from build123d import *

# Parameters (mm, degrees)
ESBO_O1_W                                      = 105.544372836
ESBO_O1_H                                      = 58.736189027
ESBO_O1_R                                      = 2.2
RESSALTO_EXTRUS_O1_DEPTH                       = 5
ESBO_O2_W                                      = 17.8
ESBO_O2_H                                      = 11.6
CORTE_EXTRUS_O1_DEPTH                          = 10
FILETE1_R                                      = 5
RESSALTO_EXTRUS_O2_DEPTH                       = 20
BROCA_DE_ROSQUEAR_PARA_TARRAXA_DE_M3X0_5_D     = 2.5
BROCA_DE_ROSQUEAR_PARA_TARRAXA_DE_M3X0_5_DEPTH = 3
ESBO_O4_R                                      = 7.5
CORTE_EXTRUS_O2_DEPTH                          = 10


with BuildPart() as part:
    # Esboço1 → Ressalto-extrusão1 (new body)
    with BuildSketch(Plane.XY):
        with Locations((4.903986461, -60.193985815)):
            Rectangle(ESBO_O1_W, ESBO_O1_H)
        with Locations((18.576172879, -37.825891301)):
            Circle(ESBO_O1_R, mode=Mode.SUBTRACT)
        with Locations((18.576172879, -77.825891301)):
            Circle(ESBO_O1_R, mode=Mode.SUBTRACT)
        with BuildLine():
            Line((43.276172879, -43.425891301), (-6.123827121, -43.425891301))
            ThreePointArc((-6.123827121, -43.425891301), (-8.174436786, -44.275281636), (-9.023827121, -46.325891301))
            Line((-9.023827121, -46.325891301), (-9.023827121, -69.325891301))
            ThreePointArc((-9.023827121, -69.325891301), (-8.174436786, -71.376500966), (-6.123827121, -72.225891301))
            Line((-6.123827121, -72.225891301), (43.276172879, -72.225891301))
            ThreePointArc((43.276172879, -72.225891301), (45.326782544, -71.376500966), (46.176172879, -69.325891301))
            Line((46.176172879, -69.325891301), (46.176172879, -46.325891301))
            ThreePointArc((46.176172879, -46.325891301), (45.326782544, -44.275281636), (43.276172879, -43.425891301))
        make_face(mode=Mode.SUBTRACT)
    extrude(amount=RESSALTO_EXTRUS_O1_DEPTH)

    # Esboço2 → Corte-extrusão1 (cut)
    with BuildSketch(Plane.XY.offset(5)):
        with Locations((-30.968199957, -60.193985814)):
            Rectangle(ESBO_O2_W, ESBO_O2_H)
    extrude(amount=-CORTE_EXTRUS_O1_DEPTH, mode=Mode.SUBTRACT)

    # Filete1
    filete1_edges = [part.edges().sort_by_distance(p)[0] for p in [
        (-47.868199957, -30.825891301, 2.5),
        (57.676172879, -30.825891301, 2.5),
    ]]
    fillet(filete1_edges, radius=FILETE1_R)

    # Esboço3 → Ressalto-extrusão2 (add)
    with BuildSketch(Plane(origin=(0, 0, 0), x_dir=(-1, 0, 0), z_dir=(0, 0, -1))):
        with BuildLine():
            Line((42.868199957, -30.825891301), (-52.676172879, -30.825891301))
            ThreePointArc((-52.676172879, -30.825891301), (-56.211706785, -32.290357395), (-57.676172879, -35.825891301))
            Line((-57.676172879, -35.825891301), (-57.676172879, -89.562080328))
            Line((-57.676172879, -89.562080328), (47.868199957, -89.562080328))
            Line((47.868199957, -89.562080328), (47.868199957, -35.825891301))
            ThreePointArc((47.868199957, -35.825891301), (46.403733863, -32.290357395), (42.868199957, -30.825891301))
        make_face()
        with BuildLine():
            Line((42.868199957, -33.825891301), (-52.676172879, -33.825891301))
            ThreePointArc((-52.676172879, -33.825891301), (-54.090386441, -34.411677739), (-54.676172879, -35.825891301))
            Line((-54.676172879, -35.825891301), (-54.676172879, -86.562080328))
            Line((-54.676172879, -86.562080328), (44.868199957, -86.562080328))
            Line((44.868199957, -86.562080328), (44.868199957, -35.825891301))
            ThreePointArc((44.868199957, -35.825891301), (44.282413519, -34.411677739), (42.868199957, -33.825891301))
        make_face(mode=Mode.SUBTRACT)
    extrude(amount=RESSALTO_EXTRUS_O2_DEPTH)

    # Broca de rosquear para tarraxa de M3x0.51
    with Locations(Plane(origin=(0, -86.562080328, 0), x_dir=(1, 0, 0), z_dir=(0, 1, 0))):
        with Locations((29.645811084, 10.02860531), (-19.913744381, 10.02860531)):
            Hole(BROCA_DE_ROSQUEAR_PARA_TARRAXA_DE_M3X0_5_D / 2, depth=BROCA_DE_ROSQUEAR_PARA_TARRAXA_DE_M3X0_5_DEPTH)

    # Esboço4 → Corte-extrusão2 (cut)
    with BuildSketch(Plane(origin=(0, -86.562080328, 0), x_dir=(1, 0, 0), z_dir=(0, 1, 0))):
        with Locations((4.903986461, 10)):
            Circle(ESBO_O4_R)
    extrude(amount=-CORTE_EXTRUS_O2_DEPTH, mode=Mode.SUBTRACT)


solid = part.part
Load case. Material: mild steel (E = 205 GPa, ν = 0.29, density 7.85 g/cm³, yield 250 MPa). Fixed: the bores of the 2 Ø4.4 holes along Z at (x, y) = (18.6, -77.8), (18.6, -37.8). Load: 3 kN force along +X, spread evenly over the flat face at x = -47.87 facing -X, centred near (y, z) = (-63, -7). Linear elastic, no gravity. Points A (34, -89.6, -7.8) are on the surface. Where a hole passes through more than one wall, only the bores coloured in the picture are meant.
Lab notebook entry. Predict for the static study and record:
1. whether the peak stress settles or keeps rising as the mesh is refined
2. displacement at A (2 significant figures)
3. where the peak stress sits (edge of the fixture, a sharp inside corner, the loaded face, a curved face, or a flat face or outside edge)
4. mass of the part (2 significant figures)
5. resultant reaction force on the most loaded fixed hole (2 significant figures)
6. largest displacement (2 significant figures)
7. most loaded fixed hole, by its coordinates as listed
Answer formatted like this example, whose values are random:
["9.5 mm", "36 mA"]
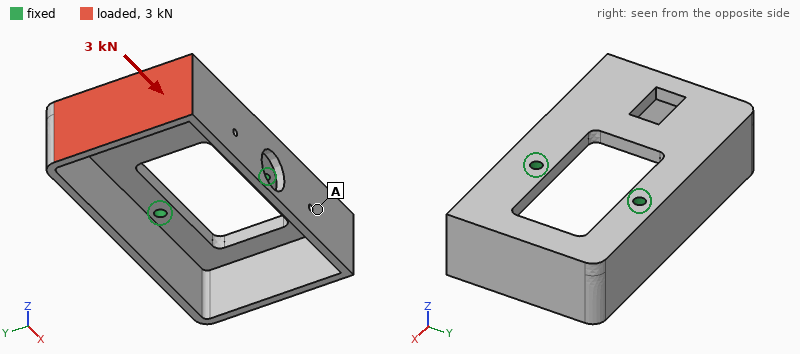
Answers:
["keeps rising", "0.032 mm", "edge of the fixture", "310 g", "1.8 kN", "0.18 mm", "(18.6, -77.8)"]
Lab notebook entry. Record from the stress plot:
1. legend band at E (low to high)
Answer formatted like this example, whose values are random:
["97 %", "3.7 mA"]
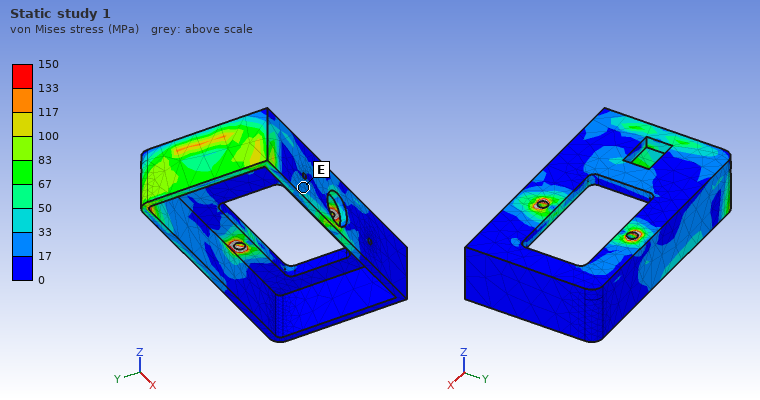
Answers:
["17 to 33 MPa"]
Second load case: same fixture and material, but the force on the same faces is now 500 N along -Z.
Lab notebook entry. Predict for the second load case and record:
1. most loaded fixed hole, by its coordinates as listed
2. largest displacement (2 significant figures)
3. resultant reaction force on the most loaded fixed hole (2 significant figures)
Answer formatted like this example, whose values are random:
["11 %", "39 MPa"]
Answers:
["(18.6, -77.8)", "0.16 mm", "280 N"]
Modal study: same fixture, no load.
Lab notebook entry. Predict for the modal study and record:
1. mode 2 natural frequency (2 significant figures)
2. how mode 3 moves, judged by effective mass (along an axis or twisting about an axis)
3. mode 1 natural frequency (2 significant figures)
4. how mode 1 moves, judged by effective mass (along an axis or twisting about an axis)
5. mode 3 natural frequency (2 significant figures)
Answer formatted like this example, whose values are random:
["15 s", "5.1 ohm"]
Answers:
["1600 Hz", "along Y", "970 Hz", "along Z", "3000 Hz"]
